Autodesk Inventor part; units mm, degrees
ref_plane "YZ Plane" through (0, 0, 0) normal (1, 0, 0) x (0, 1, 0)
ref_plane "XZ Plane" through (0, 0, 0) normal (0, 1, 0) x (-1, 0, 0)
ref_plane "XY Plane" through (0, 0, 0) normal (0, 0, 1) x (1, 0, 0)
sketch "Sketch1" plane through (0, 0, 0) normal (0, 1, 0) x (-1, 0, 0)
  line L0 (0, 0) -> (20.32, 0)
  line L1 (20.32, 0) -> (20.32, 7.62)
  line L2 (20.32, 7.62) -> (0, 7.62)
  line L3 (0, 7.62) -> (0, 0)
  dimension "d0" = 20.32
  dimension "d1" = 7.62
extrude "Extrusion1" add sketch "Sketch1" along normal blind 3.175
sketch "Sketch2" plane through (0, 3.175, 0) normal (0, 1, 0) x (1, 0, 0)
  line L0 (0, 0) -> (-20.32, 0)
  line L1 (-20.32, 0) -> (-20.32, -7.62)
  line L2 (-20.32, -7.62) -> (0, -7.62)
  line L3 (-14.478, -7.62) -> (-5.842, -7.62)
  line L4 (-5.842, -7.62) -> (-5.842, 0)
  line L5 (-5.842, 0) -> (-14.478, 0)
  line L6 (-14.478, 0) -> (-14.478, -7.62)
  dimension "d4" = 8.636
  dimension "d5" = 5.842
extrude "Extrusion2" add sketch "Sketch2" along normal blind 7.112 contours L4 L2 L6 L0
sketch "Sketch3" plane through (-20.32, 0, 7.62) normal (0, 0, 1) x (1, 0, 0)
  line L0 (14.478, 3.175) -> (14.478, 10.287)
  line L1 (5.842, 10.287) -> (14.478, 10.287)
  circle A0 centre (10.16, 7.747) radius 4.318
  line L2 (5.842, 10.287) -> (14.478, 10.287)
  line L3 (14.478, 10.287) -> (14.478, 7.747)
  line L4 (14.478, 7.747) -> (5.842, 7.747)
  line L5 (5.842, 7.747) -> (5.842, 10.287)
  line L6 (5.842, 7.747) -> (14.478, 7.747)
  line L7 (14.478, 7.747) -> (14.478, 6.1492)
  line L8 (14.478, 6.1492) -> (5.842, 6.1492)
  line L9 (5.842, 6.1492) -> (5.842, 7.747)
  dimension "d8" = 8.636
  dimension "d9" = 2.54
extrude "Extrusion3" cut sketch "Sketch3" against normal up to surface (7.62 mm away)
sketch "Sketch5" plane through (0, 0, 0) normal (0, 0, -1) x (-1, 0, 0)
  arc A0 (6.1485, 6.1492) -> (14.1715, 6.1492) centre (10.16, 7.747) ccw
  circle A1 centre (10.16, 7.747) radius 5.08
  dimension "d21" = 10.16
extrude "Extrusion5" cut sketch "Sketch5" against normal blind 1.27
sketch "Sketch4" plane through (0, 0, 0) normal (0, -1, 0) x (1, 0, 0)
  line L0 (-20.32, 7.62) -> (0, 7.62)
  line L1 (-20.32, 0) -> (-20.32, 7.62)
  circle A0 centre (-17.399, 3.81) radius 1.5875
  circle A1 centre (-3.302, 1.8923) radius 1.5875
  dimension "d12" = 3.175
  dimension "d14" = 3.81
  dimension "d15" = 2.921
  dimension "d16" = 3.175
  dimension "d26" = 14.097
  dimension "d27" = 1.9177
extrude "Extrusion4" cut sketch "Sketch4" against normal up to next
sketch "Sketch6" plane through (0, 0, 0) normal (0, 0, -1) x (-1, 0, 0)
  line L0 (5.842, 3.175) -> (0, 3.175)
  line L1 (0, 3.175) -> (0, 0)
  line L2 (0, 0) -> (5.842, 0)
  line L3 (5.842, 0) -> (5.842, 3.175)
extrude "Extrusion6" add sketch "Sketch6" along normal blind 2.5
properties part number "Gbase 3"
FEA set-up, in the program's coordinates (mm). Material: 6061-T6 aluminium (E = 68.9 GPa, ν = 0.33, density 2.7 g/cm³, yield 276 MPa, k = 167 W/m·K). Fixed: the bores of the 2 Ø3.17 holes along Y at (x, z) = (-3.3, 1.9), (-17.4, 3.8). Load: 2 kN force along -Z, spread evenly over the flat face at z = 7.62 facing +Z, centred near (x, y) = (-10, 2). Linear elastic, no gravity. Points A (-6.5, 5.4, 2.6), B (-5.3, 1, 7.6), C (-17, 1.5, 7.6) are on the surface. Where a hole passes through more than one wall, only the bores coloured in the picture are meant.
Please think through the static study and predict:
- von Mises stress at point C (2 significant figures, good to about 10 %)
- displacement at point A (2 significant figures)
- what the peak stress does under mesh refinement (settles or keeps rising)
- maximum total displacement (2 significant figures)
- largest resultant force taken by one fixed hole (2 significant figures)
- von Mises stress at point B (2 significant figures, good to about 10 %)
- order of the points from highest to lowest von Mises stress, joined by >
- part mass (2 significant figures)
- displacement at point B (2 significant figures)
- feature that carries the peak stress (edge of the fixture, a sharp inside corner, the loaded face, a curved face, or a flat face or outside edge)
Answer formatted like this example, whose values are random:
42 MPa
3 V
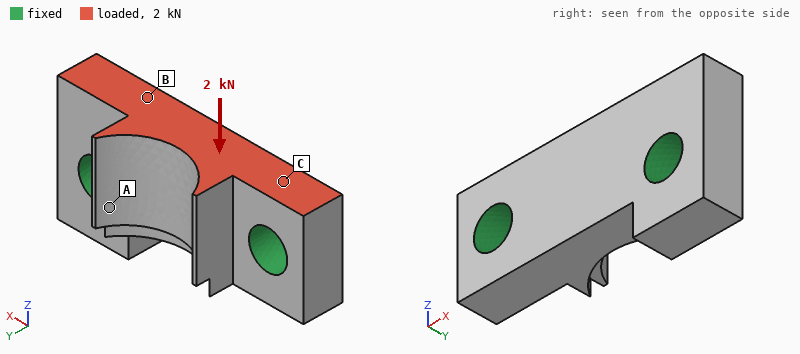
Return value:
47 MPa
5.3 µm
keeps rising
7.9 µm
1.1 kN
28 MPa
C > B > A
1.5 g
4.0 µm
edge of the fixture
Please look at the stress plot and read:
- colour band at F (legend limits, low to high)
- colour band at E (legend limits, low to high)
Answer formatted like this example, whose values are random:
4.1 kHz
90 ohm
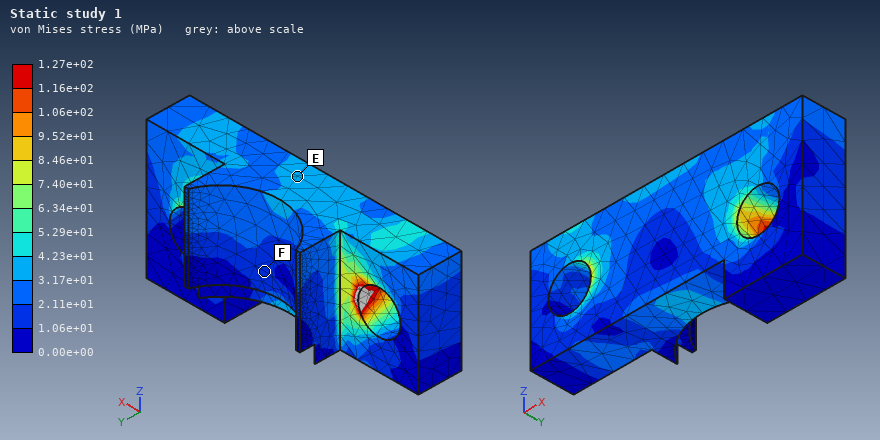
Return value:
1.06e+01 to 2.11e+01 MPa
3.17e+01 to 4.23e+01 MPa
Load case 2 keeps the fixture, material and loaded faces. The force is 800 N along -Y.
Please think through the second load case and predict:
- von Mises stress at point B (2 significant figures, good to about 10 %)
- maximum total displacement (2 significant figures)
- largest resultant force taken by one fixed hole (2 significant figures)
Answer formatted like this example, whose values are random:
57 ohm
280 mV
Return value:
28 MPa
18 µm
420 N
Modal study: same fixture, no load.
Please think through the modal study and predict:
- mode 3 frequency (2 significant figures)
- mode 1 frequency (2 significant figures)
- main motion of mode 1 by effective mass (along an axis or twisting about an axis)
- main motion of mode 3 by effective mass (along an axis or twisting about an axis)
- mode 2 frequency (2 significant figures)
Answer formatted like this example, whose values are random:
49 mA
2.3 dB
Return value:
89 kHz
62 kHz
along Y
along Z
81 kHz
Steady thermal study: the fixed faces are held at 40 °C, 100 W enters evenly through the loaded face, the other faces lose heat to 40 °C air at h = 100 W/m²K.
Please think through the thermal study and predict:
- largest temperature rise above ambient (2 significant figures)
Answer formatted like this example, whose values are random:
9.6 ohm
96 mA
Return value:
54 K
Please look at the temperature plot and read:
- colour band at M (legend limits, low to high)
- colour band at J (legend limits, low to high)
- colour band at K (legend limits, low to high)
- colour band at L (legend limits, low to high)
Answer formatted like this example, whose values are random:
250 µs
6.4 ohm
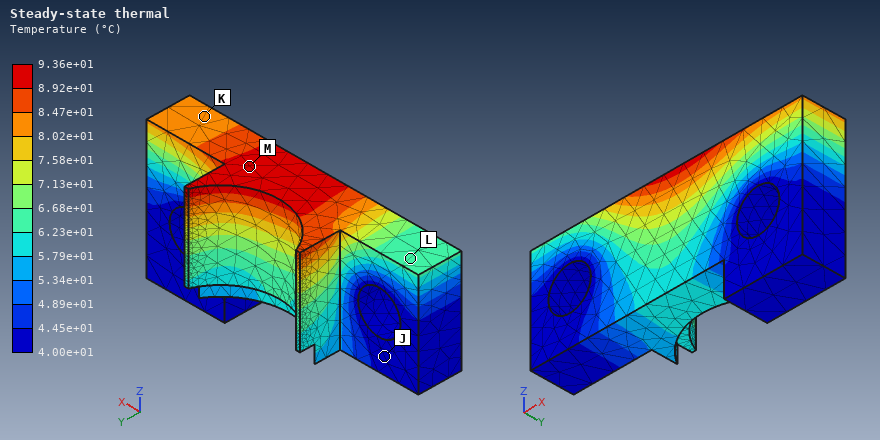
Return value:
8.92e+01 to 9.36e+01 °C
4.00e+01 to 4.45e+01 °C
8.02e+01 to 8.47e+01 °C
6.23e+01 to 6.68e+01 °C
